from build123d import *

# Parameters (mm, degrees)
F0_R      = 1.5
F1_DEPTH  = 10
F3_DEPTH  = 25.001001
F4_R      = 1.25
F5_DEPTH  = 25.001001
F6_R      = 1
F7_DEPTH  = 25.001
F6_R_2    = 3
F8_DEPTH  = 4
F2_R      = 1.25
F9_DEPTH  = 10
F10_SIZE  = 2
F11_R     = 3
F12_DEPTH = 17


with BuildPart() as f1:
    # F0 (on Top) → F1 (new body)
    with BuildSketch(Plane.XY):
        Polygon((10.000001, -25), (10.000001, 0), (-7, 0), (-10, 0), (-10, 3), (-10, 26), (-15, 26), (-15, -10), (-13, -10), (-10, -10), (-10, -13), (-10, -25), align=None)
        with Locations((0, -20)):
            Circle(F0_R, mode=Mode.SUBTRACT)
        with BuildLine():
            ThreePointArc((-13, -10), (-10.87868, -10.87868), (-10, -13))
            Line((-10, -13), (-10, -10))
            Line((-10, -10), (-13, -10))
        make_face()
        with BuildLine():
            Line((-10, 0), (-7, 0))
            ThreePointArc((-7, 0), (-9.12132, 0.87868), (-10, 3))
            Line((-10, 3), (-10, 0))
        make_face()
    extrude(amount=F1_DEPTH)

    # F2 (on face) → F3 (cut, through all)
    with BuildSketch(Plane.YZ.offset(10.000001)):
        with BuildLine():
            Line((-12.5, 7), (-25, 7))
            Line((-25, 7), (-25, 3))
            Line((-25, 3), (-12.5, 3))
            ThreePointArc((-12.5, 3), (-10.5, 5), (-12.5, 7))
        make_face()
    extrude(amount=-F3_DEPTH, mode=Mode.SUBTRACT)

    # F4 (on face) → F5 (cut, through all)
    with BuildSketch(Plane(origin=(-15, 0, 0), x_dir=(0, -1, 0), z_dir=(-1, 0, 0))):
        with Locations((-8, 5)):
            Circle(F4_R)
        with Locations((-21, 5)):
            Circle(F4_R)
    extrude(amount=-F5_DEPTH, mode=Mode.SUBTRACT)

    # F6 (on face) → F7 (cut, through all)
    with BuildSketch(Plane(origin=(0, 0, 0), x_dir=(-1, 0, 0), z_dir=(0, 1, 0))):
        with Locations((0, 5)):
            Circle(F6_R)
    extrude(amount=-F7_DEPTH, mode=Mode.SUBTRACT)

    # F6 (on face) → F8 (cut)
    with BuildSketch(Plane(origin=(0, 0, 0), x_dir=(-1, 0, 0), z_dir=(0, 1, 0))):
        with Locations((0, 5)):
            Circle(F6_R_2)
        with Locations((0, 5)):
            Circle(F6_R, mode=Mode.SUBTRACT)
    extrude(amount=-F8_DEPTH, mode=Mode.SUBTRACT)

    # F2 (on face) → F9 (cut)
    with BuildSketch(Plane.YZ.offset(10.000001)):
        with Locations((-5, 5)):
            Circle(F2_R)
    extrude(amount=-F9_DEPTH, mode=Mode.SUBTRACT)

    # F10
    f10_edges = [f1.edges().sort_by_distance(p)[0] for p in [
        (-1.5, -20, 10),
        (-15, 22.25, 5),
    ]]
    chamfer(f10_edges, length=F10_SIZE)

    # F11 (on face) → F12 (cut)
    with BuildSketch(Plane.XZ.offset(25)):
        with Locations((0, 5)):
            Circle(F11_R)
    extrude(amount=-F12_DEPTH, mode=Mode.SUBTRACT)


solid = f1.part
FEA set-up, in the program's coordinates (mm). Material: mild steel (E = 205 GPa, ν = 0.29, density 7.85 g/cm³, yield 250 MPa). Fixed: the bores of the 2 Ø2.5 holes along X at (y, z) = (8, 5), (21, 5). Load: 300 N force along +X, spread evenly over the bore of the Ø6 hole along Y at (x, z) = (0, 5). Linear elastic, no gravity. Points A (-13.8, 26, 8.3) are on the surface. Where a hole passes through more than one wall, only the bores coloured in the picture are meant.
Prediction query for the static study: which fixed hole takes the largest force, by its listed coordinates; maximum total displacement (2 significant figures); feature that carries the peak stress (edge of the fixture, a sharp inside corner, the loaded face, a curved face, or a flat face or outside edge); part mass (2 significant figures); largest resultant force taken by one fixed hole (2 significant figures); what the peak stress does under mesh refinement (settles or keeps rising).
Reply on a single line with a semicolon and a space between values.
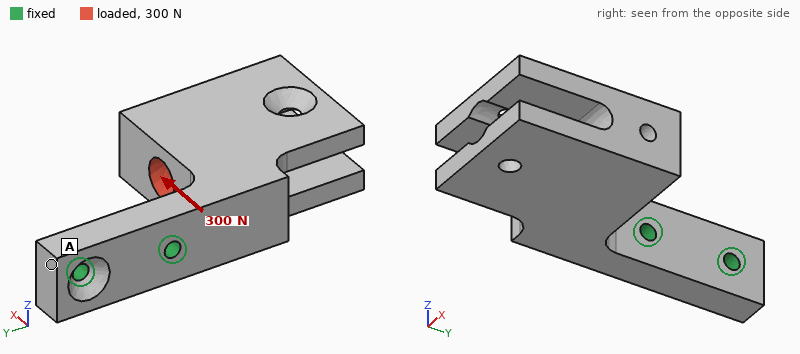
(8, 5); 26 µm; edge of the fixture; 41 g; 340 N; keeps rising
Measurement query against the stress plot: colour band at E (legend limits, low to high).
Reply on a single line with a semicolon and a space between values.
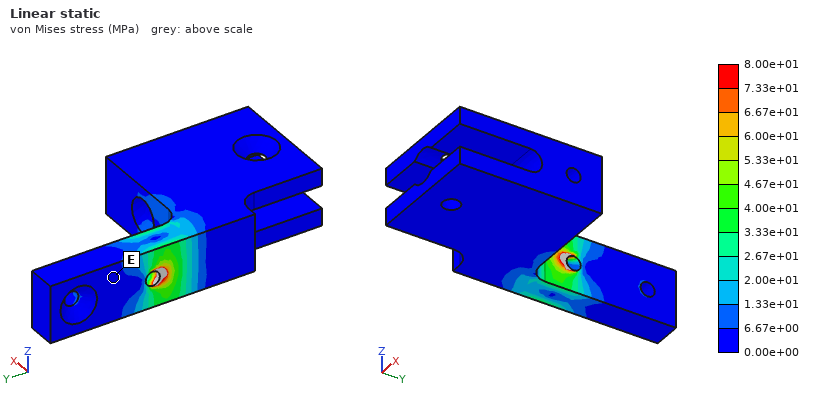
0.00e+00 to 6.67e+00 MPa
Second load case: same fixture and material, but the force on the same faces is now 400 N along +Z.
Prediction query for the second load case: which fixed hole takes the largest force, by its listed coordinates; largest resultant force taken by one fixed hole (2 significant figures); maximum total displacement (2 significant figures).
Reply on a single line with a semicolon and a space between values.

(8, 5); 580 N; 51 µm
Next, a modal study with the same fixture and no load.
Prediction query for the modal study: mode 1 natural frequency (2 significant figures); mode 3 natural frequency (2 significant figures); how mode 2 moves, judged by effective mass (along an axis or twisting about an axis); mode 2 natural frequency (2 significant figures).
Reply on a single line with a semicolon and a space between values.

2100 Hz; 6500 Hz; along Z; 2800 Hz
